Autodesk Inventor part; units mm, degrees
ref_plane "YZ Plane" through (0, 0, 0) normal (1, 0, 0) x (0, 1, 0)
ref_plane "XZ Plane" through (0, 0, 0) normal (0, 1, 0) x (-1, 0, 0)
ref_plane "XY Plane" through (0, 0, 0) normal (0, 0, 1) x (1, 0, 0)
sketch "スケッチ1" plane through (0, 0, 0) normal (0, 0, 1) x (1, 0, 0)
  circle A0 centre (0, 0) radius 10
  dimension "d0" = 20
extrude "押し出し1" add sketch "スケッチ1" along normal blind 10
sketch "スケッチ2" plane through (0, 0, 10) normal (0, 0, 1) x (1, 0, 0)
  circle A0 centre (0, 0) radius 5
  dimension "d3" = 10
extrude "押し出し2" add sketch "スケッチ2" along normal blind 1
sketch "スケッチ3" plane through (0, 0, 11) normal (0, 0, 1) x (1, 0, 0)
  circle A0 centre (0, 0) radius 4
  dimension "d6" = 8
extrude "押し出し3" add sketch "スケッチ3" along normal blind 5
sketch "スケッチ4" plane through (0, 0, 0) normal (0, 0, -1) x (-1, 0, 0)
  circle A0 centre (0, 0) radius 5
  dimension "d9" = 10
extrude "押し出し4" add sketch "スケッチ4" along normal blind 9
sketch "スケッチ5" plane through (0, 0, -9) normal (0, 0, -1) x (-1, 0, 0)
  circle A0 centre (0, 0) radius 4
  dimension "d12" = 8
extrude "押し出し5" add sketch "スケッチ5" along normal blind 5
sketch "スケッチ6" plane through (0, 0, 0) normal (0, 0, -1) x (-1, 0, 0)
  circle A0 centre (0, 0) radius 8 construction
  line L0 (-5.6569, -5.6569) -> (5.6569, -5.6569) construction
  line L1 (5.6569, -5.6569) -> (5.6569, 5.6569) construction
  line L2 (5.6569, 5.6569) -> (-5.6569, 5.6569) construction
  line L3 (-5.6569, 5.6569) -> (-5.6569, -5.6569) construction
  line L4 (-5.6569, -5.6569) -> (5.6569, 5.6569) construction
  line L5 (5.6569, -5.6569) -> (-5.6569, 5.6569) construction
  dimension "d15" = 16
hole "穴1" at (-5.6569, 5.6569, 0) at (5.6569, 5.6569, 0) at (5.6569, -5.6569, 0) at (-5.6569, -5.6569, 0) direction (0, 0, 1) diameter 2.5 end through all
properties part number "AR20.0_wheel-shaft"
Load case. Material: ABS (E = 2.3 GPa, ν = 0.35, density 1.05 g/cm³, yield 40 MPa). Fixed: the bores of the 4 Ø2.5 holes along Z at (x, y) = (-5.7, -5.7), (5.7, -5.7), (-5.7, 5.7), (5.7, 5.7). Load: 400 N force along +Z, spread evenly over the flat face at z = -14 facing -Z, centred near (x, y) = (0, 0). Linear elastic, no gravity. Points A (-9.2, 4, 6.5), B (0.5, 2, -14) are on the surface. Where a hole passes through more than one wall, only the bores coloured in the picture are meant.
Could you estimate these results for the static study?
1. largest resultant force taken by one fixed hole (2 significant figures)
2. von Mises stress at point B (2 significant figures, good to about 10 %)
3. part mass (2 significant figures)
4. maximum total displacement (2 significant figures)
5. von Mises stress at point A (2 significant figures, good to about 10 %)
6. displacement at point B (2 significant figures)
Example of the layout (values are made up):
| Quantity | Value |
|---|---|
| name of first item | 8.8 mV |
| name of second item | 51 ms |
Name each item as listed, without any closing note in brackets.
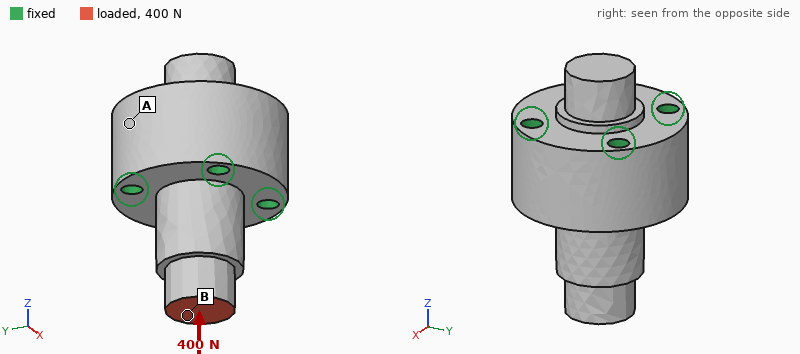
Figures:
| Quantity | Value |
|---|---|
| largest resultant force taken by one fixed hole | 110 N |
| von Mises stress at point B | 8.1 MPa |
| part mass | 4.4 g |
| maximum total displacement | 49 µm |
| von Mises stress at point A | 0.81 MPa |
| displacement at point B | 48 µm |
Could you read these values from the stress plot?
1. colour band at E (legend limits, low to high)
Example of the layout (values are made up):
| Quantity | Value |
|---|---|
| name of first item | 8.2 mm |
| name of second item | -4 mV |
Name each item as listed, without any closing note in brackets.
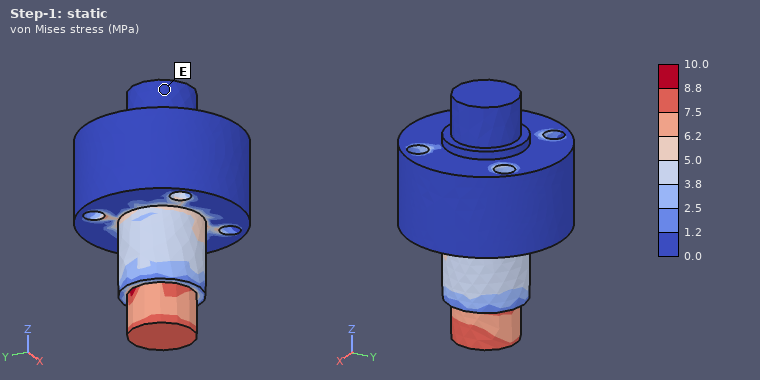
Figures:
| Quantity | Value |
|---|---|
| colour band at E | 0.0 to 1.2 MPa |
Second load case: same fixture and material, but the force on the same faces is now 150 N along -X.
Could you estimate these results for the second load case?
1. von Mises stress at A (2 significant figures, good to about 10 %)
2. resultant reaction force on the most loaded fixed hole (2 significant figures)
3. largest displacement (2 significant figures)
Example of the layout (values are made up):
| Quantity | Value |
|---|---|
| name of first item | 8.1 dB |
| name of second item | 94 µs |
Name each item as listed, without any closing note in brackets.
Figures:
| Quantity | Value |
|---|---|
| von Mises stress at A | 1.8 MPa |
| resultant reaction force on the most loaded fixed hole | 110 N |
| largest displacement | 0.25 mm |
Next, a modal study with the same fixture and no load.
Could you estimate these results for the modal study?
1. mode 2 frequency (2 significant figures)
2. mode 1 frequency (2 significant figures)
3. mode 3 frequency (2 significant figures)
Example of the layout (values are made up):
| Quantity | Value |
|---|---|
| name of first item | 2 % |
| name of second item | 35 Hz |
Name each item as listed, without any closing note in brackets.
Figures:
| Quantity | Value |
|---|---|
| mode 2 frequency | 8000 Hz |
| mode 1 frequency | 7900 Hz |
| mode 3 frequency | 18 kHz |
